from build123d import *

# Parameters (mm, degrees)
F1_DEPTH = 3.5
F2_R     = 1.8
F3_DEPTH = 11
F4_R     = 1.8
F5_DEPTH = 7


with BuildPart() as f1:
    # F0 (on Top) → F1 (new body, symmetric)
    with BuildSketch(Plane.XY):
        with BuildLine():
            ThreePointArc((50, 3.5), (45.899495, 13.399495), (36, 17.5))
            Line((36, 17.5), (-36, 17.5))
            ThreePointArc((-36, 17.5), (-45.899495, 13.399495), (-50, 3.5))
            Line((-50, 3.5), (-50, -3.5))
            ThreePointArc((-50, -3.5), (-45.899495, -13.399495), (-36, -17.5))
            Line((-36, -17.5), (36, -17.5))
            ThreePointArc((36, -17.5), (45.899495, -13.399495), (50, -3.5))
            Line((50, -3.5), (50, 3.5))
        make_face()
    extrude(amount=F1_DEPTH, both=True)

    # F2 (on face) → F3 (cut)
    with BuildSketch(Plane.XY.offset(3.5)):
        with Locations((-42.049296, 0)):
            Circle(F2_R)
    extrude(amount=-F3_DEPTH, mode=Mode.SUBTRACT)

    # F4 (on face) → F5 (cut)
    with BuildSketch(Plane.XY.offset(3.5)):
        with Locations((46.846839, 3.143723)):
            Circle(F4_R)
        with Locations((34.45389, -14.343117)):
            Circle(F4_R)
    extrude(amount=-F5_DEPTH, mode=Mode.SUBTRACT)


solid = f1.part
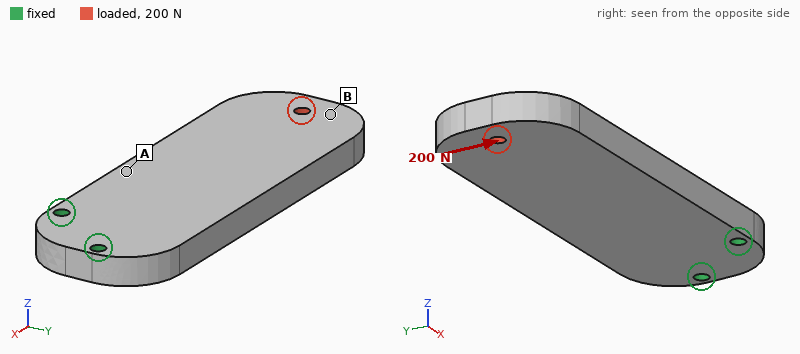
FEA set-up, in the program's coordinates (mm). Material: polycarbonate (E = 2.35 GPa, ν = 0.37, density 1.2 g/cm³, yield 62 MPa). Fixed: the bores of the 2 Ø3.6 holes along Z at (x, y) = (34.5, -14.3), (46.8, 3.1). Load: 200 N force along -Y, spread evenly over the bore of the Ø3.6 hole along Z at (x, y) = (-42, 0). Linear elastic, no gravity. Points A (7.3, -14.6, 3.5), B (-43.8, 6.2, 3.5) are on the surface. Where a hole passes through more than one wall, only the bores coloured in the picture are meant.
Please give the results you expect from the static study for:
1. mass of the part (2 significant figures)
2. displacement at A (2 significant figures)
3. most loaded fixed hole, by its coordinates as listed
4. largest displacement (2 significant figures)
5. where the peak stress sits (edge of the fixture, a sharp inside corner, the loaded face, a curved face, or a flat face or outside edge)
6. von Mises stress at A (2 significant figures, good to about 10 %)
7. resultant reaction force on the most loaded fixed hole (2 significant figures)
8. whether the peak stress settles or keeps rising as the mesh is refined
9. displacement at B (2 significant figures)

28 g
0.24 mm
(34.5, -14.3)
0.96 mm
edge of the fixture
5.7 MPa
770 N
keeps rising
0.89 mm
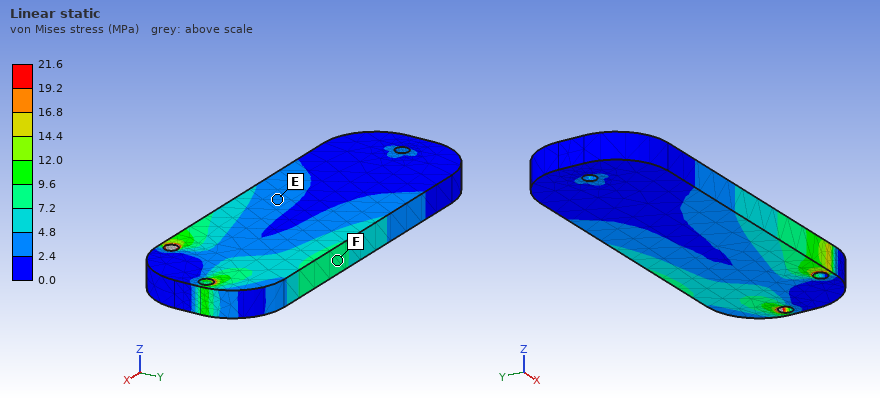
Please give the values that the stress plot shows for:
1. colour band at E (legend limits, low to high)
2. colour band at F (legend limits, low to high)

2.4 to 4.8 MPa
7.2 to 9.6 MPa
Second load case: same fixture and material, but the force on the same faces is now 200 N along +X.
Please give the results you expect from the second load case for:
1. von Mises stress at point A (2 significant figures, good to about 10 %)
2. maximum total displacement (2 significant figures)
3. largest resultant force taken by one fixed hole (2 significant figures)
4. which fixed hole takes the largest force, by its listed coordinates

0.83 MPa
60 µm
140 N
(46.8, 3.1)
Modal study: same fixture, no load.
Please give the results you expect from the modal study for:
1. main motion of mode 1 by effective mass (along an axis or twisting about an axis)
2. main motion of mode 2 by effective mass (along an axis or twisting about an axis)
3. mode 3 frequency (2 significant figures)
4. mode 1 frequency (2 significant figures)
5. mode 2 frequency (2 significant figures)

along Z
along Y
920 Hz
210 Hz
830 Hz
